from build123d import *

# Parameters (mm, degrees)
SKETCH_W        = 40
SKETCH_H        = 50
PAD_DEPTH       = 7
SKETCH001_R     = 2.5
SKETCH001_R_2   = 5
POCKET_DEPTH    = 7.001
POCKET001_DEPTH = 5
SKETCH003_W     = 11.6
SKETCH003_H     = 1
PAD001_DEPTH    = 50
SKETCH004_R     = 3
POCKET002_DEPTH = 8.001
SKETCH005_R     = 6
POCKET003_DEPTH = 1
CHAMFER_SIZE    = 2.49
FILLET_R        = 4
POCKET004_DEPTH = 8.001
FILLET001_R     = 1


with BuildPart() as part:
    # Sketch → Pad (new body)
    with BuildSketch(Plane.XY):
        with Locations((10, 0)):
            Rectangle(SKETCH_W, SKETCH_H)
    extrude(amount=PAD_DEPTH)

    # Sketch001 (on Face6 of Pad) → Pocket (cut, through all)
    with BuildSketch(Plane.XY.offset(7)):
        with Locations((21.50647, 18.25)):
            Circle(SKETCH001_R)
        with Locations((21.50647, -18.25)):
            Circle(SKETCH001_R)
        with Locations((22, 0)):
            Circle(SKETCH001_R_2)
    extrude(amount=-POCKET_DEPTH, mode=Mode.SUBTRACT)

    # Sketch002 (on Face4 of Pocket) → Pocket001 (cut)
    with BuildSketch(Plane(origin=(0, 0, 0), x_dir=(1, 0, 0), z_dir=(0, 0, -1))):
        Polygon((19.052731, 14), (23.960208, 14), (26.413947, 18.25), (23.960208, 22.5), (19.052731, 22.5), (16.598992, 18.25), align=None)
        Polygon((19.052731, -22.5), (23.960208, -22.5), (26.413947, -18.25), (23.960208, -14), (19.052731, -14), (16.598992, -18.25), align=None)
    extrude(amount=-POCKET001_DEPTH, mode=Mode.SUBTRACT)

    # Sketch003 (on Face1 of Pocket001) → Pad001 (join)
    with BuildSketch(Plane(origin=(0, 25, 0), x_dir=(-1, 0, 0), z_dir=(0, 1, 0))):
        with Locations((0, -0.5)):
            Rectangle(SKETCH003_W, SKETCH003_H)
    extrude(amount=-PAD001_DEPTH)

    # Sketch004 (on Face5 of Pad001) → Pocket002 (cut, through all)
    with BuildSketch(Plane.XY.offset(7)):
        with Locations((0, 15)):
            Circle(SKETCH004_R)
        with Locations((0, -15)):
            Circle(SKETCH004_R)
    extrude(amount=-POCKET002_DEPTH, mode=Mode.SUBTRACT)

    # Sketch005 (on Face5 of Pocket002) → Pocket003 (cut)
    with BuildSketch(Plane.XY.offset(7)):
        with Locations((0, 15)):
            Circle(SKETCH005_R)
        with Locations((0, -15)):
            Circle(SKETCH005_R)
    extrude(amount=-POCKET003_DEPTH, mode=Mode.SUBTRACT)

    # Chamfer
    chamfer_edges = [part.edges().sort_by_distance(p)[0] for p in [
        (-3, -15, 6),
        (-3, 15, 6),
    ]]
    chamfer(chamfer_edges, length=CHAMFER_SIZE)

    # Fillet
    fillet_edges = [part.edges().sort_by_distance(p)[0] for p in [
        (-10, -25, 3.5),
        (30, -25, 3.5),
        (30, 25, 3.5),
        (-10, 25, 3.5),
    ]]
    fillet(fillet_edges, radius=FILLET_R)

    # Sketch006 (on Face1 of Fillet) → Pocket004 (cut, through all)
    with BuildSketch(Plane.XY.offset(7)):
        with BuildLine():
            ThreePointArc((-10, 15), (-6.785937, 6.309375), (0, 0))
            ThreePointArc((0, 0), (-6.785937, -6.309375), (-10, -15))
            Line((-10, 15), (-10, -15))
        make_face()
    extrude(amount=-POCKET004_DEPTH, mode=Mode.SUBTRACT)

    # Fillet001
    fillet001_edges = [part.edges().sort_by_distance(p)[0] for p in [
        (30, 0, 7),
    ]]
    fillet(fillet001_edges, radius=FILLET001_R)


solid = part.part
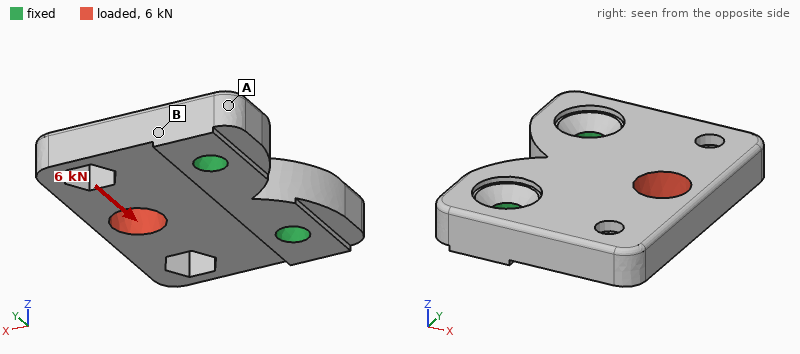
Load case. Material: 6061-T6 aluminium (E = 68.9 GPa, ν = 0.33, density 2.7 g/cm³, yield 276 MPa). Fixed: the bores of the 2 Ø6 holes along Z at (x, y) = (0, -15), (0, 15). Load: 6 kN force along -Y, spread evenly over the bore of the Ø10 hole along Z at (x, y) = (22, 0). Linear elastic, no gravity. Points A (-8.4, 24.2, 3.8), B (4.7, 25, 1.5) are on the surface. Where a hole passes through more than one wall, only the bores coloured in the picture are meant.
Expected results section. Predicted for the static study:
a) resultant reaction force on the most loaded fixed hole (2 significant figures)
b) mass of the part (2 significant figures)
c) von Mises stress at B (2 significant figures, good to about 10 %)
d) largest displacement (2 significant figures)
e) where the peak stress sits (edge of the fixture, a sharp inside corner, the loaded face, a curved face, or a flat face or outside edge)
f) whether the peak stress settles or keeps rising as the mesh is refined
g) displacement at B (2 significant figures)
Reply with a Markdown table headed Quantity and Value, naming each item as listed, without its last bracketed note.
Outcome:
| Quantity | Value |
|---|---|
| resultant reaction force on the most loaded fixed hole | 4.8 kN |
| mass of the part | 32 g |
| von Mises stress at B | 30 MPa |
| largest displacement | 46 µm |
| where the peak stress sits | edge of the fixture |
| whether the peak stress settles or keeps rising as the mesh is refined | keeps rising |
| displacement at B | 12 µm |
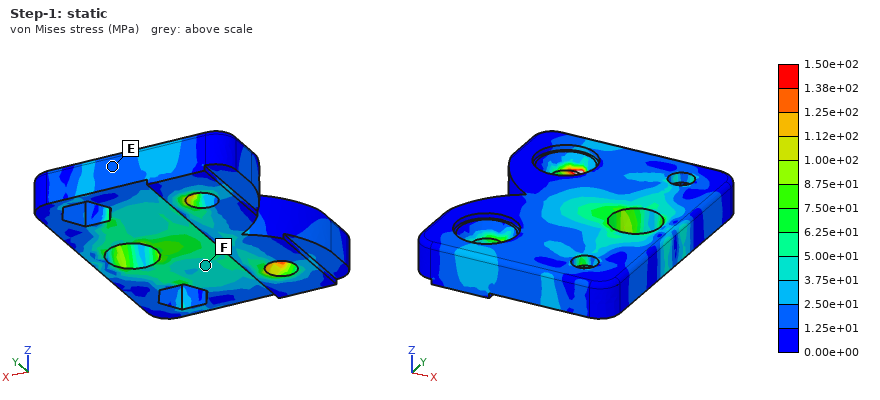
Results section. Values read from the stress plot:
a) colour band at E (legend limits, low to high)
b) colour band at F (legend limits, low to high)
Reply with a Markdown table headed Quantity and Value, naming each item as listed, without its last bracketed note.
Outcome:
| Quantity | Value |
|---|---|
| colour band at E | 1.25e+01 to 2.50e+01 MPa |
| colour band at F | 3.75e+01 to 5.00e+01 MPa |
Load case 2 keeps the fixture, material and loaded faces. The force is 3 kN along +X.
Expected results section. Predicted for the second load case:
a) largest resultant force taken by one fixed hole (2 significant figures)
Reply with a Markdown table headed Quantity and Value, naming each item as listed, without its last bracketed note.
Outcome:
| Quantity | Value |
|---|---|
| largest resultant force taken by one fixed hole | 1.6 kN |
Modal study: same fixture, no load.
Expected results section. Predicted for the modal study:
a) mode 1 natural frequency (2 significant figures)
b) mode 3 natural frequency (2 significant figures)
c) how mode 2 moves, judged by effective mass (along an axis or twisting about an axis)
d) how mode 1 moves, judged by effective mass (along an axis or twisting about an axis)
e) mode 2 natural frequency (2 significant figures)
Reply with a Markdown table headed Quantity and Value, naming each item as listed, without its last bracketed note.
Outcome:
| Quantity | Value |
|---|---|
| mode 1 natural frequency | 5700 Hz |
| mode 3 natural frequency | 18 kHz |
| how mode 2 moves, judged by effective mass | twisting about X |
| how mode 1 moves, judged by effective mass | along Z |
| mode 2 natural frequency | 9400 Hz |
